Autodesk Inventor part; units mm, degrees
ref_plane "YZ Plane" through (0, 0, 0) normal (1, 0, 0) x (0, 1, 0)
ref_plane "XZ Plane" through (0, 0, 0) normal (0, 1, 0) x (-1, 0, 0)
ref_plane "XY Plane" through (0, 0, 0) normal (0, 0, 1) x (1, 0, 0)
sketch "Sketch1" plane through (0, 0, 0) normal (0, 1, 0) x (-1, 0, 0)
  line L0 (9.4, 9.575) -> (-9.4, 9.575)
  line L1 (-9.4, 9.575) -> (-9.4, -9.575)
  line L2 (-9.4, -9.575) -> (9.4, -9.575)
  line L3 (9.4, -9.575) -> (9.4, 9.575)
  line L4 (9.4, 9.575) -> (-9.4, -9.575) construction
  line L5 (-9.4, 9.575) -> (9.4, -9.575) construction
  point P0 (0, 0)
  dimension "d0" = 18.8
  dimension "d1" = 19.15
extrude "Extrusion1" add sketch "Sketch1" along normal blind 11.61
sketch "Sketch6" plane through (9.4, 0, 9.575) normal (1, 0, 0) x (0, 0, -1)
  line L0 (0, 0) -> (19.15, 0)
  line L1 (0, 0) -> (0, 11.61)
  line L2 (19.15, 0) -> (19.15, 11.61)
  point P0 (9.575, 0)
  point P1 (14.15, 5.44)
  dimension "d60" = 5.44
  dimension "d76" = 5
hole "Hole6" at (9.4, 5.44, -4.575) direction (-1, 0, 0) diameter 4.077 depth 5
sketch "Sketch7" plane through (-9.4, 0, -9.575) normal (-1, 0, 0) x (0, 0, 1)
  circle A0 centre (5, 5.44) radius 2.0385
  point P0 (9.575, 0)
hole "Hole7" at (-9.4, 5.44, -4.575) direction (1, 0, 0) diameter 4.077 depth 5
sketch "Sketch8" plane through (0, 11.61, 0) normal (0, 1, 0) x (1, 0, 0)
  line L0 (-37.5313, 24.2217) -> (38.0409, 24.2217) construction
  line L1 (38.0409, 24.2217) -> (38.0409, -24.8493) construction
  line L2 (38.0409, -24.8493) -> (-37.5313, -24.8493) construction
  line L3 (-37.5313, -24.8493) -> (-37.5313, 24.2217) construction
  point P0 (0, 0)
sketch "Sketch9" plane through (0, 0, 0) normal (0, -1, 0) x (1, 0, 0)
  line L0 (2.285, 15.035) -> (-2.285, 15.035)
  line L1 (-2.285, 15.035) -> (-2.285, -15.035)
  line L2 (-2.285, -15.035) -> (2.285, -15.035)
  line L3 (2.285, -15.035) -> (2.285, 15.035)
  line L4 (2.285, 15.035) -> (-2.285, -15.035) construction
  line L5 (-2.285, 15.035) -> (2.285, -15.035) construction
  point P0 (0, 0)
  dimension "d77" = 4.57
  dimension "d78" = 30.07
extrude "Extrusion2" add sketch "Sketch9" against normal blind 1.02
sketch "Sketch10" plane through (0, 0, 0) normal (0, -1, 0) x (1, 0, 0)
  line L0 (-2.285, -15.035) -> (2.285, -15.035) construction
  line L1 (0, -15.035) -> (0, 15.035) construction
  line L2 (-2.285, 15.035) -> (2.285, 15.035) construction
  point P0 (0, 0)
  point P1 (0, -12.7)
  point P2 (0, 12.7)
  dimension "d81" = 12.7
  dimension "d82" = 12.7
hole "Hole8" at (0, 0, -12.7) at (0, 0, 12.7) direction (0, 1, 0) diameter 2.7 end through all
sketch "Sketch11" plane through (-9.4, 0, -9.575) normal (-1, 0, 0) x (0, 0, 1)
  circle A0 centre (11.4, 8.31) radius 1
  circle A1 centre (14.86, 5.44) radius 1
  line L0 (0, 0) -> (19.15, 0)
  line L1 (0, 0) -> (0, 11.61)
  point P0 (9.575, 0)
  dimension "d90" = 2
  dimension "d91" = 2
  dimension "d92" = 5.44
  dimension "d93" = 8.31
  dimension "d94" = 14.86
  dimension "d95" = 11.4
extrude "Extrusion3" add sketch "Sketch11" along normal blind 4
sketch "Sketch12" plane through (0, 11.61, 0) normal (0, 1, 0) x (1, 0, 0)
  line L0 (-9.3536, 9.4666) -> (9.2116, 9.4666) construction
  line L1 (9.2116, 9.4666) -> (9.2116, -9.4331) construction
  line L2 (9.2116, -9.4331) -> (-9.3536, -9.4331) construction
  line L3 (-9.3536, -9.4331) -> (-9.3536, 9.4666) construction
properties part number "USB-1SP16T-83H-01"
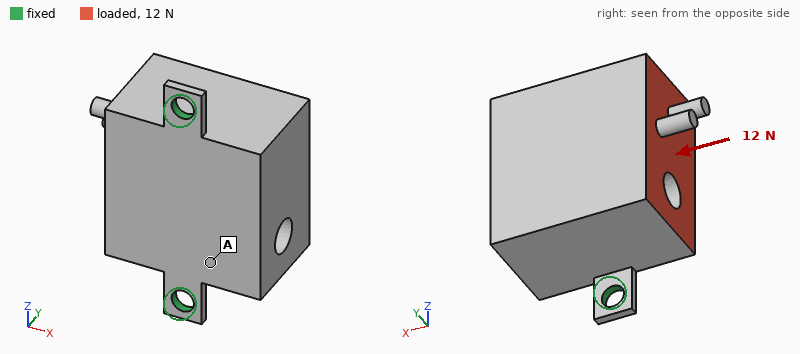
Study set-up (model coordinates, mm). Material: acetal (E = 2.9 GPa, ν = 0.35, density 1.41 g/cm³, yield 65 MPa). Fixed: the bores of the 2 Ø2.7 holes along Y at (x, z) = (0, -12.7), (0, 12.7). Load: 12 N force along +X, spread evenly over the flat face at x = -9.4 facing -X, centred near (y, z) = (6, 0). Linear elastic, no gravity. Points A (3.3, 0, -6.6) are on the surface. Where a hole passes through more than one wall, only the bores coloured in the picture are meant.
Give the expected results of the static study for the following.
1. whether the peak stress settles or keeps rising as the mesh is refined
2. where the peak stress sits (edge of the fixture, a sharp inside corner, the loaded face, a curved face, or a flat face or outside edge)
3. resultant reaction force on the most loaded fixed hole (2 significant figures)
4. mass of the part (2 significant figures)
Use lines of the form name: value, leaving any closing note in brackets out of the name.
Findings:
whether the peak stress settles or keeps rising as the mesh is refined: keeps rising
where the peak stress sits: edge of the fixture
resultant reaction force on the most loaded fixed hole: 6.1 N
mass of the part: 5.8 g
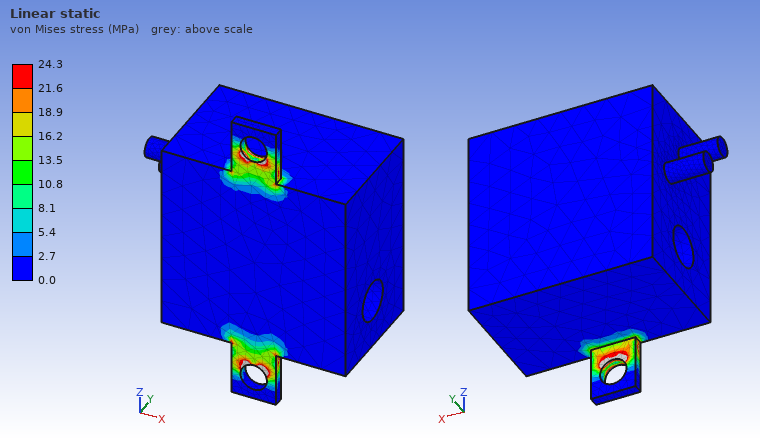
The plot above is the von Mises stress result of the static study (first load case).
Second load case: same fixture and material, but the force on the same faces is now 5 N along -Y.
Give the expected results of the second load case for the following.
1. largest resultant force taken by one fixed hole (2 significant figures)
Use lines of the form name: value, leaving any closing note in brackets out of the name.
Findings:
largest resultant force taken by one fixed hole: 2.9 N
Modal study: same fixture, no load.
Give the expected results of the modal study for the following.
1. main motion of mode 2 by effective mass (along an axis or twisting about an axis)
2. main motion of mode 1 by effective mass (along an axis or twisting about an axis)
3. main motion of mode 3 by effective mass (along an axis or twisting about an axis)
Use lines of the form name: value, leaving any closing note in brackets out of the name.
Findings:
main motion of mode 2 by effective mass: along Y
main motion of mode 1 by effective mass: along X
main motion of mode 3 by effective mass: along Z
